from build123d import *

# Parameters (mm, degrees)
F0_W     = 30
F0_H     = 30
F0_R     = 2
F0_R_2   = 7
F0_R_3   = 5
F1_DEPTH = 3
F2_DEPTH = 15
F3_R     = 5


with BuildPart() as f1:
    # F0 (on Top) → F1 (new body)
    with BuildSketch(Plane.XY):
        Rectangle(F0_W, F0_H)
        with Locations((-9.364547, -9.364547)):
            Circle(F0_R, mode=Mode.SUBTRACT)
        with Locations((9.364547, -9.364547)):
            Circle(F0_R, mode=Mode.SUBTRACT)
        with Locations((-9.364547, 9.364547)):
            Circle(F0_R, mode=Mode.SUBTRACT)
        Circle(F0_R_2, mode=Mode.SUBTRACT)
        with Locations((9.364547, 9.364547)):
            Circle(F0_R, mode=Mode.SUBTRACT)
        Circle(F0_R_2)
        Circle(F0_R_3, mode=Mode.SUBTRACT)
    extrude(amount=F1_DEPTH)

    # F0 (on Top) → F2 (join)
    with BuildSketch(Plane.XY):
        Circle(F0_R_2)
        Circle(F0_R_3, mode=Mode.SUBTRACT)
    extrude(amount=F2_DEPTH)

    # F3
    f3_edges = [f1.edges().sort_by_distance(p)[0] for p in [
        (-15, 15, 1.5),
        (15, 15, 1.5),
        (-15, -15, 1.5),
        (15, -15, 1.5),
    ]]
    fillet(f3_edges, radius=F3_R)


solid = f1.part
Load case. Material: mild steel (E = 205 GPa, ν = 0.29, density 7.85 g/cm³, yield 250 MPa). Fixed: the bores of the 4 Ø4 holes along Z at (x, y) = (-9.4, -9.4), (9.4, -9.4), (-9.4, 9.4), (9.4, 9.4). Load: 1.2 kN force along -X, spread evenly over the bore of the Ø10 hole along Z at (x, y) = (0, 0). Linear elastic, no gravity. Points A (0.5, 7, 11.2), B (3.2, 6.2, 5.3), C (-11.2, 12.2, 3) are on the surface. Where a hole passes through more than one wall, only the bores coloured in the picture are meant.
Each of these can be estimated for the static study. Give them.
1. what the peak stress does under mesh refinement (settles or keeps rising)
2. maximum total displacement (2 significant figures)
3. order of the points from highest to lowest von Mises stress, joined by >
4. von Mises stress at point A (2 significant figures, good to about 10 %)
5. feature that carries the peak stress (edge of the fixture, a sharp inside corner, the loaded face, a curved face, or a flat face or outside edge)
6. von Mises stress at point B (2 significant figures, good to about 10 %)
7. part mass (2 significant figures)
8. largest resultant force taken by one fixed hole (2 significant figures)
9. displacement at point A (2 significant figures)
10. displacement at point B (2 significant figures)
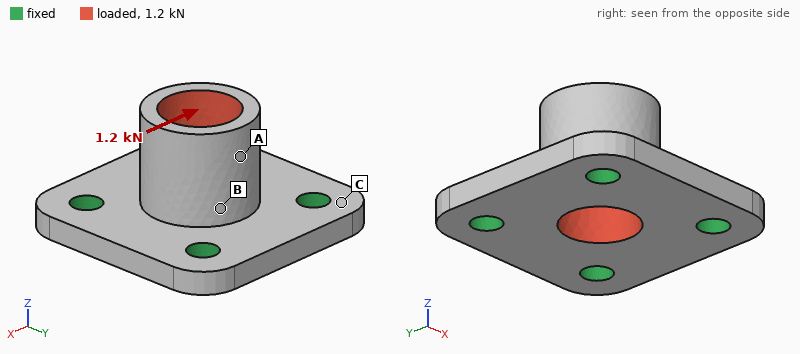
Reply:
keeps rising
7.8 µm
B > A > C
11 MPa
edge of the fixture
22 MPa
25 g
400 N
5.2 µm
2.3 µm
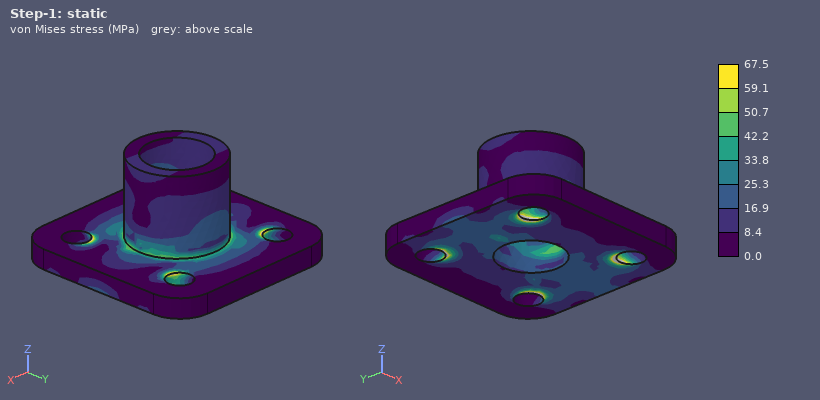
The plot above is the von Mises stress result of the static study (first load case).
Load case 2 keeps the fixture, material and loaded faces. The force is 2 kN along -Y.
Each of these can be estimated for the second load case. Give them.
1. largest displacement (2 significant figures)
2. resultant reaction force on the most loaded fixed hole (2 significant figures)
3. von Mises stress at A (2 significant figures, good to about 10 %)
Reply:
13 µm
660 N
14 MPa
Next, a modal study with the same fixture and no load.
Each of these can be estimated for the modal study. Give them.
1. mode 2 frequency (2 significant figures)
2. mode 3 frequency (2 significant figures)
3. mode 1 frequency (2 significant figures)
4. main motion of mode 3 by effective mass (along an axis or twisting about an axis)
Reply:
23 kHz
31 kHz
23 kHz
along Z
